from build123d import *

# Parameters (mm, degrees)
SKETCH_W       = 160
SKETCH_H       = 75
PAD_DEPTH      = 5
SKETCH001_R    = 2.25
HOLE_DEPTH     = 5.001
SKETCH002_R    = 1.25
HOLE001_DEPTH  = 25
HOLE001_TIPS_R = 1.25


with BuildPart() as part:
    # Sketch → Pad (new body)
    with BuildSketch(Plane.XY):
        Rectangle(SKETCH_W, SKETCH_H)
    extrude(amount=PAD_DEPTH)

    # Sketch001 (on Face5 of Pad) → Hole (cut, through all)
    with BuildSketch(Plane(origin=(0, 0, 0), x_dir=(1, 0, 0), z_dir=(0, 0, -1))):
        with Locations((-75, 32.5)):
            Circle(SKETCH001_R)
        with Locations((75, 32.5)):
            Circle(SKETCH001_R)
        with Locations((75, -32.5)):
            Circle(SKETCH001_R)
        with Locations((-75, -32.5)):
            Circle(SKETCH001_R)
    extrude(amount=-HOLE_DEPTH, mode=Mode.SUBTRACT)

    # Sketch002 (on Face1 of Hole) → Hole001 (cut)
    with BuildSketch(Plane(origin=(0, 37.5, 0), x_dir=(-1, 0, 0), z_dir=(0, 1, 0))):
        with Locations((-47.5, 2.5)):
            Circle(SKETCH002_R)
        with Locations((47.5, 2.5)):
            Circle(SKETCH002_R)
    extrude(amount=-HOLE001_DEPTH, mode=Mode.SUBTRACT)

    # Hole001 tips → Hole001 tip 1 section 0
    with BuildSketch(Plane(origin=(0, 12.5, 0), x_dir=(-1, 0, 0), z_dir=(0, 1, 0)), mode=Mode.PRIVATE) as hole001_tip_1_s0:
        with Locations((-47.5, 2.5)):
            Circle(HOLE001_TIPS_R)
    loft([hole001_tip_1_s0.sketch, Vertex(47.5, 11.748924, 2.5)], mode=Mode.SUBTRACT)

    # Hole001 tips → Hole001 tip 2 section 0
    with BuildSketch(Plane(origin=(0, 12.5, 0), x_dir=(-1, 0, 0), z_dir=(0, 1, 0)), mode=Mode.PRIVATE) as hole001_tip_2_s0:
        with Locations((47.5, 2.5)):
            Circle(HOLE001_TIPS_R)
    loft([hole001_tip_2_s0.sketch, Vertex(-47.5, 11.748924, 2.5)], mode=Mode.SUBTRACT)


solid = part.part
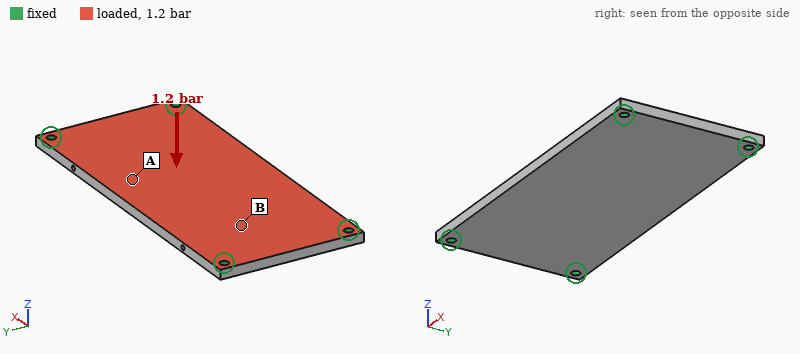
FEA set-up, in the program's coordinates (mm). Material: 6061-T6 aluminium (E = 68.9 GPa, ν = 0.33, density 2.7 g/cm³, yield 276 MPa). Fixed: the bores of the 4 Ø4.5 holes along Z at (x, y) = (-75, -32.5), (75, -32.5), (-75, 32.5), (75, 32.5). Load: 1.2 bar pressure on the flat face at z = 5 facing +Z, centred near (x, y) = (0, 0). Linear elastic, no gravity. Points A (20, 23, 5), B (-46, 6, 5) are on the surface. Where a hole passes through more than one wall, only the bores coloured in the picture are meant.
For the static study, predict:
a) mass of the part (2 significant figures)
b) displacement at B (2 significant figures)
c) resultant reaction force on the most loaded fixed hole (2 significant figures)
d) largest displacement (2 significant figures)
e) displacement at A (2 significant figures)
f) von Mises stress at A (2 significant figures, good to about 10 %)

160 g
0.15 mm
360 N
0.32 mm
0.27 mm
26 MPa
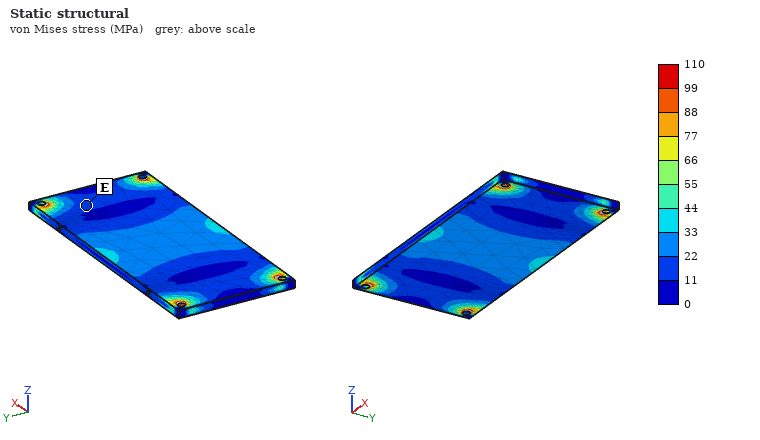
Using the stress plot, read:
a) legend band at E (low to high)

11 to 22 MPa
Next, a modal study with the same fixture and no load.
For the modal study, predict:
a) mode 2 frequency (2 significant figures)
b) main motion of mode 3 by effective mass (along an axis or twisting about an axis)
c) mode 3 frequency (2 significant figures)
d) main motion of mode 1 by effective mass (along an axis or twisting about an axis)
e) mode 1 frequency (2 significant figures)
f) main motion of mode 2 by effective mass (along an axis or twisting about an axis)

1900 Hz
twisting about Y
2700 Hz
along Z
980 Hz
twisting about X
